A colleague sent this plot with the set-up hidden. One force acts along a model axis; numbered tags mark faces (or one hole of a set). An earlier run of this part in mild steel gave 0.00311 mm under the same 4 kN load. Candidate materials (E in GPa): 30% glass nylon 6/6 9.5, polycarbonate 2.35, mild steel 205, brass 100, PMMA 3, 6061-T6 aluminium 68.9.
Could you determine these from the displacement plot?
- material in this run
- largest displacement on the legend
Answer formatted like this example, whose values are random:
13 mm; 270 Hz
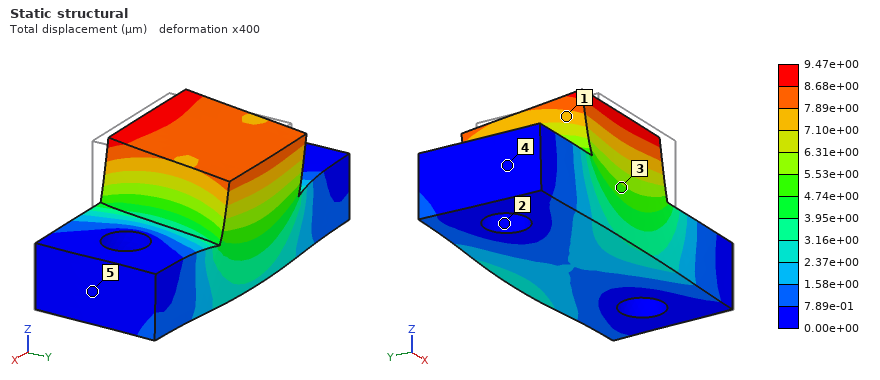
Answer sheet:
6061-T6 aluminium; 9.47e+00 µm
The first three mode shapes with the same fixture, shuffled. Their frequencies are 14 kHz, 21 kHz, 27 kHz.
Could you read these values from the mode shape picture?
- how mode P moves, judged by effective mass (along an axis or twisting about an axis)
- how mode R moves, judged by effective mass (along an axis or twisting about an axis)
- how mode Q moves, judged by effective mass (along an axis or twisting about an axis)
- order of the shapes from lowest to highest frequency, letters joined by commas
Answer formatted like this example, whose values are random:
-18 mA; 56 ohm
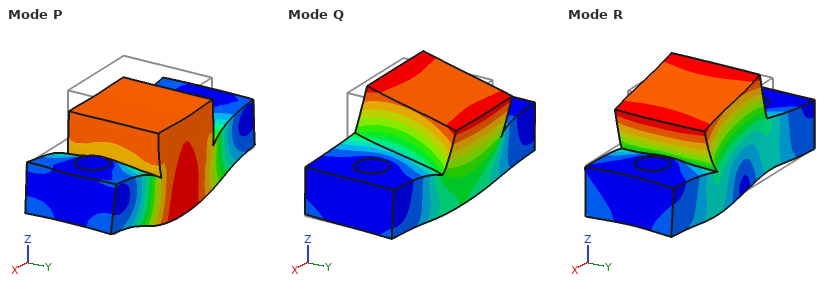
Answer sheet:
along Z; along X; along Y; Q, P, R
